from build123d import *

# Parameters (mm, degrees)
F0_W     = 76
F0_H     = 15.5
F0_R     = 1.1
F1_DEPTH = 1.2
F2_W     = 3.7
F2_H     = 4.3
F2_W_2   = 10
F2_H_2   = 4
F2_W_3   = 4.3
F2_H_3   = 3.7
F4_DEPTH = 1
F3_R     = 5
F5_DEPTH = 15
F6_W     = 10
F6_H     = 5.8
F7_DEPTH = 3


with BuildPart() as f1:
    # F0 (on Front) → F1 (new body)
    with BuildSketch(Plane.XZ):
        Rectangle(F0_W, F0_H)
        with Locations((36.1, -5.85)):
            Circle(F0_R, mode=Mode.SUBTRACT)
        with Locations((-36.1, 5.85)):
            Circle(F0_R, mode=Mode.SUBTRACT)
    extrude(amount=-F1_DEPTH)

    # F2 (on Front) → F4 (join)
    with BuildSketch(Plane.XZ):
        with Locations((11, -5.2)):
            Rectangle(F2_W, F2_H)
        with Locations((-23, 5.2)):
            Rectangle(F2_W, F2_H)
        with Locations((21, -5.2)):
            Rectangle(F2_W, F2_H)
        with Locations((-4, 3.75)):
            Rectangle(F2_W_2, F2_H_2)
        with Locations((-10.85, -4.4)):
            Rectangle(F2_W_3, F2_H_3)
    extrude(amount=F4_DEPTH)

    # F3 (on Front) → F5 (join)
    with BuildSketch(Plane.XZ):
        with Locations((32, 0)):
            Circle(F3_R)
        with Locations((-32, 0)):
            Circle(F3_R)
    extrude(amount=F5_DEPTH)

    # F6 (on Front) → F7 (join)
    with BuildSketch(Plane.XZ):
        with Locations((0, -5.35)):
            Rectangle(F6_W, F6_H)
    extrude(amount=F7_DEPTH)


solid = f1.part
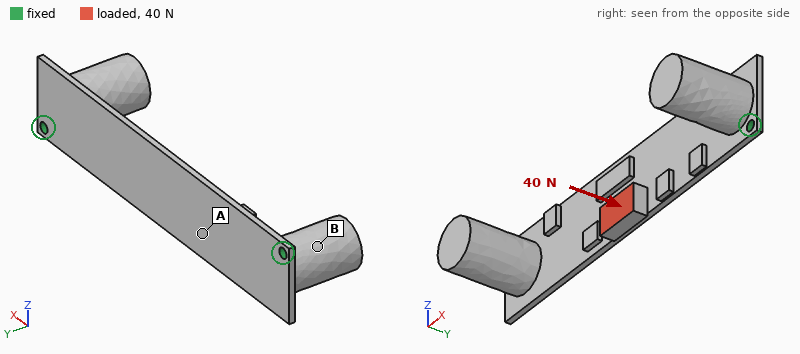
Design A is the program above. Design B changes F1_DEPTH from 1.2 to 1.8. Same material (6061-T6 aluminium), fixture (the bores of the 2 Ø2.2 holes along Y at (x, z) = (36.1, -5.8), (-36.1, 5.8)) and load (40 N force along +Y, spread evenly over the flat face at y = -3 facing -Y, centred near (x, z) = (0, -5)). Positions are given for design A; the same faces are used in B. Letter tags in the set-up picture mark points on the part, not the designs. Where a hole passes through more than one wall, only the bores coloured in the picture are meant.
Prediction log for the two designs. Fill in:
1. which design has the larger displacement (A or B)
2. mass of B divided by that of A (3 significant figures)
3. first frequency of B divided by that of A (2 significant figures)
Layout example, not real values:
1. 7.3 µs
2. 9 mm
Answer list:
1. A
2. 1.17
3. 1.5
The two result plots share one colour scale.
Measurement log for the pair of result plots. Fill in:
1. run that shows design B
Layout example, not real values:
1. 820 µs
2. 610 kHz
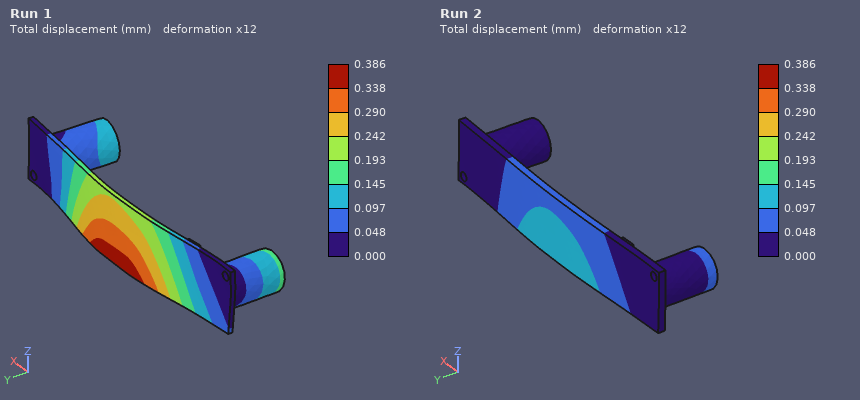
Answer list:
1. Run 2
